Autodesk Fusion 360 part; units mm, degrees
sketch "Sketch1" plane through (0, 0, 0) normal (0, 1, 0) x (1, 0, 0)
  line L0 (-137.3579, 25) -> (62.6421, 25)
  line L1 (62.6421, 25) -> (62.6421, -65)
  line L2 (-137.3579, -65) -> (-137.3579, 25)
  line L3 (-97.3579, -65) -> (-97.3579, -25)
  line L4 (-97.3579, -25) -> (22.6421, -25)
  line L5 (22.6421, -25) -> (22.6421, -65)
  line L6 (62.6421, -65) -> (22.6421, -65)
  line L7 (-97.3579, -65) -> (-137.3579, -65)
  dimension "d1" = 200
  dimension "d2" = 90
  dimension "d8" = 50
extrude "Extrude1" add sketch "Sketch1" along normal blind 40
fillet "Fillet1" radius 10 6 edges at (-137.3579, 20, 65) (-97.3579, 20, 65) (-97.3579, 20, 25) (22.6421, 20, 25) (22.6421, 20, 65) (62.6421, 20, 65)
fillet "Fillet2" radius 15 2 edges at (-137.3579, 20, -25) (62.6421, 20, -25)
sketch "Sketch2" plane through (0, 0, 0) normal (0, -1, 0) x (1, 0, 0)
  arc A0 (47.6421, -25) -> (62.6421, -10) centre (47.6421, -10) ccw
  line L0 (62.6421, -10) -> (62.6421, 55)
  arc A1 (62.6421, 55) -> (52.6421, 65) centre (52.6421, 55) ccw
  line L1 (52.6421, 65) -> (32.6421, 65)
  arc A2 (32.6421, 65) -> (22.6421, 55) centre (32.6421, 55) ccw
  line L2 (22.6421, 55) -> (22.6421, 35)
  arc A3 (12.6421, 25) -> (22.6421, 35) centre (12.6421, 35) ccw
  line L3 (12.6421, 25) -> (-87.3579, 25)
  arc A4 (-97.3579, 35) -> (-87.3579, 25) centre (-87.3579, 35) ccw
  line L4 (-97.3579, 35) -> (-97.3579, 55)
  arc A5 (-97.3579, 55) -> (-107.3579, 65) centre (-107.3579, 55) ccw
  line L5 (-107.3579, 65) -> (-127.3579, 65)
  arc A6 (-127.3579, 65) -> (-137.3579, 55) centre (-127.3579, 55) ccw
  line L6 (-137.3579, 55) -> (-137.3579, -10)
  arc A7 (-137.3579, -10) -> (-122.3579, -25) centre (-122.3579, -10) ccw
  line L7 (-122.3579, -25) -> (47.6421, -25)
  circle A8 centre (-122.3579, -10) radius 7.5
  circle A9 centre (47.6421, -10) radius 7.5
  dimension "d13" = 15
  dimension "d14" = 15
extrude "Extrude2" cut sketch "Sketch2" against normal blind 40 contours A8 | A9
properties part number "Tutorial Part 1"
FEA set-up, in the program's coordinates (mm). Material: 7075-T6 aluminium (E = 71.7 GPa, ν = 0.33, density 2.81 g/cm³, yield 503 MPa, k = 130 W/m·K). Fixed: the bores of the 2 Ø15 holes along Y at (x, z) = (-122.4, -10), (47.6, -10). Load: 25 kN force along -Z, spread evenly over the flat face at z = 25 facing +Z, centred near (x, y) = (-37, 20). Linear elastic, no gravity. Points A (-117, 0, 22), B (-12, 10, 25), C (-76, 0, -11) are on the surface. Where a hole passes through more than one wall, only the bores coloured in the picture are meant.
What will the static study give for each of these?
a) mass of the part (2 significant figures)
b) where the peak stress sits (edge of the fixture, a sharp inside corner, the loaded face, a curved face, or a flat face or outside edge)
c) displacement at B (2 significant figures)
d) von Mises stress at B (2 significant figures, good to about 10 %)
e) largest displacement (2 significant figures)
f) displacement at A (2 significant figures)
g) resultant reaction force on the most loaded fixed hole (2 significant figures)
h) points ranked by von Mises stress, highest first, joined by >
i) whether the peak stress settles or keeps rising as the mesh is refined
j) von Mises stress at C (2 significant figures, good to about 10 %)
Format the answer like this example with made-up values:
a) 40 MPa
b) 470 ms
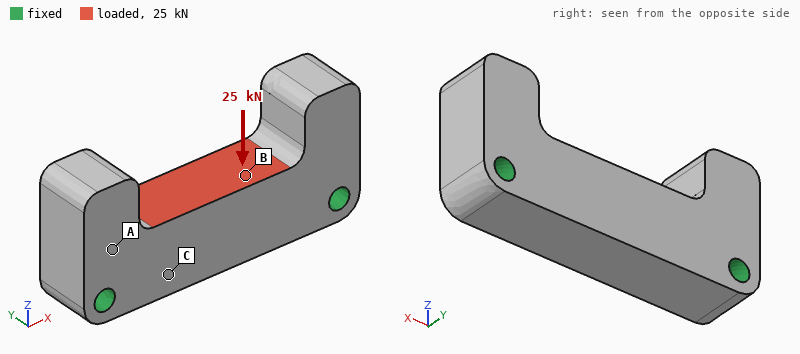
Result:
a) 1.4 kg
b) edge of the fixture
c) 38 µm
d) 22 MPa
e) 43 µm
f) 13 µm
g) 15 kN
h) B > C > A
i) keeps rising
j) 11 MPa
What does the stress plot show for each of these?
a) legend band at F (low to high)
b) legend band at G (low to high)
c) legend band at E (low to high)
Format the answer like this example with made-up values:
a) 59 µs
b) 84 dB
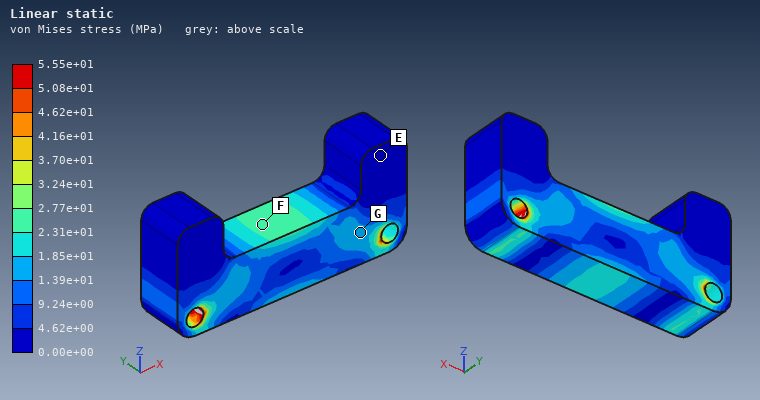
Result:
a) 2.31e+01 to 2.77e+01 MPa
b) 1.39e+01 to 1.85e+01 MPa
c) 0.00e+00 to 4.62e+00 MPa
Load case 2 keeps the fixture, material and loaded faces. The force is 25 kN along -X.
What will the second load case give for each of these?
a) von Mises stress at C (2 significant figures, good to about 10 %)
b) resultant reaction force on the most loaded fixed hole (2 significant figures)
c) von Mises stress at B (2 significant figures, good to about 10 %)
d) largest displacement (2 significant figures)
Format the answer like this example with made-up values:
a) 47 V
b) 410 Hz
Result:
a) 4.1 MPa
b) 13 kN
c) 12 MPa
d) 10 µm
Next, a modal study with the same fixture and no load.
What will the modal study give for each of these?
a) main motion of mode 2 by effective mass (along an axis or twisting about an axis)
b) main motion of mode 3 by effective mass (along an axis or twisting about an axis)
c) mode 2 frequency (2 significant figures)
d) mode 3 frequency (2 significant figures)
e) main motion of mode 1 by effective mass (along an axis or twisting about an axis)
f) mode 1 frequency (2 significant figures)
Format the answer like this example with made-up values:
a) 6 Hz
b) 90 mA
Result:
a) along Y
b) twisting about Z
c) 4700 Hz
d) 5500 Hz
e) along Z
f) 4300 Hz
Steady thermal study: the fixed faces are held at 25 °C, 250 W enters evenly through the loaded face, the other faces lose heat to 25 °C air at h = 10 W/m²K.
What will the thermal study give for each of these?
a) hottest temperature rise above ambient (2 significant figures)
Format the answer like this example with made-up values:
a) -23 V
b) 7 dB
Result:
a) 36 K
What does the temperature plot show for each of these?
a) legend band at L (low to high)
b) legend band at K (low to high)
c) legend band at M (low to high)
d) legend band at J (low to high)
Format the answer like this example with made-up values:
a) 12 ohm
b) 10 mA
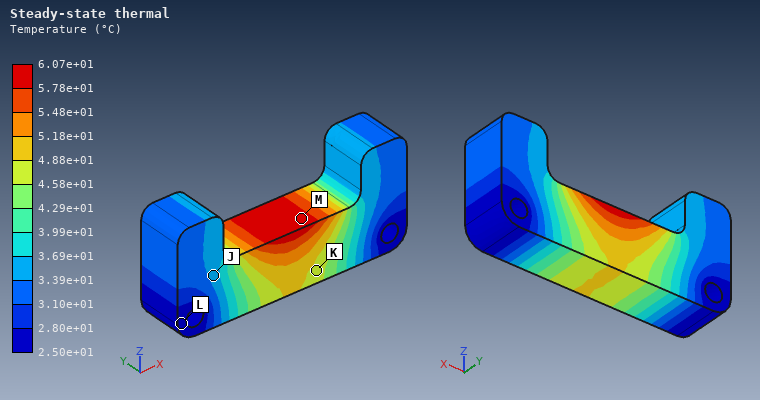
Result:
a) 2.50e+01 to 2.80e+01 °C
b) 4.58e+01 to 4.88e+01 °C
c) 5.78e+01 to 6.07e+01 °C
d) 3.39e+01 to 3.69e+01 °C
